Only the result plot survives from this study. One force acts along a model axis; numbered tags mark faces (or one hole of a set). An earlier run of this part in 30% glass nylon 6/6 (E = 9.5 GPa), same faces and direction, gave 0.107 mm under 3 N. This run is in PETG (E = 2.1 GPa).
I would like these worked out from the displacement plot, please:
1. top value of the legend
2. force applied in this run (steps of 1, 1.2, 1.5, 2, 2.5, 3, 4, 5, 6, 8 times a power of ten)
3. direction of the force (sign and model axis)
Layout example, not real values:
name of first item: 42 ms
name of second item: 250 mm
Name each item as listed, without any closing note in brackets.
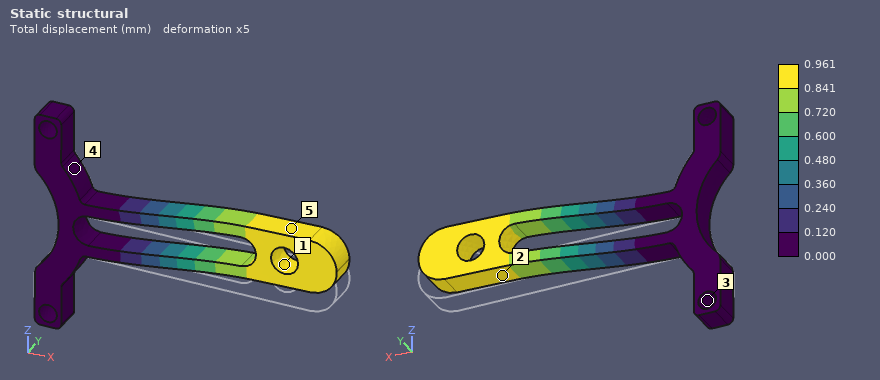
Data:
top value of the legend: 0.961 mm
force applied in this run: 6 N
direction of the force: +Z
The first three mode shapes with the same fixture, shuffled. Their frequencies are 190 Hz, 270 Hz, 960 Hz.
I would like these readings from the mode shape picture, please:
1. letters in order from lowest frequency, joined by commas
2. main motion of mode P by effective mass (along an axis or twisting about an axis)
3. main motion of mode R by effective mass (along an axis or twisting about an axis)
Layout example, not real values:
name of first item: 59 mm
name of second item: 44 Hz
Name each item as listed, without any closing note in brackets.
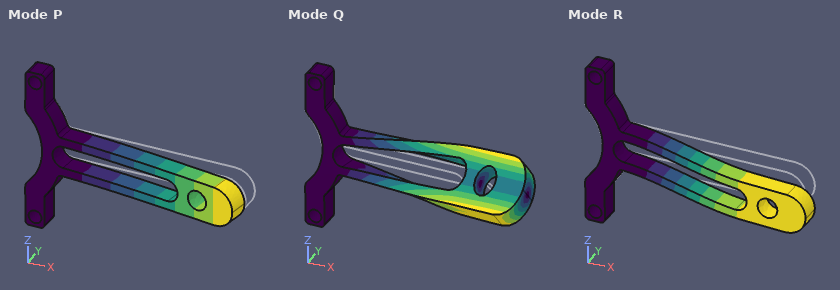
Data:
letters in order from lowest frequency, joined by commas: P, R, Q
main motion of mode P by effective mass: along Y
main motion of mode R by effective mass: along Z
